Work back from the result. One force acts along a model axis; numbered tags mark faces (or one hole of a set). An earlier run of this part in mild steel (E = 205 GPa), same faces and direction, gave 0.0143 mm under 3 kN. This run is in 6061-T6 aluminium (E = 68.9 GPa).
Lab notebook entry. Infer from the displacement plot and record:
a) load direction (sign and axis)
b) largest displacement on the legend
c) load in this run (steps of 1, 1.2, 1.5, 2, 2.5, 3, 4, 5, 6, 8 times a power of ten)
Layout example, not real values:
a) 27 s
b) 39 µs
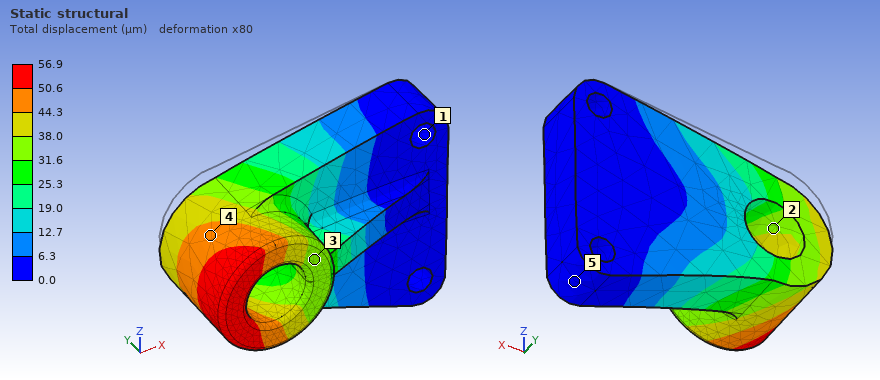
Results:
a) -Z
b) 56.9 µm
c) 4 kN
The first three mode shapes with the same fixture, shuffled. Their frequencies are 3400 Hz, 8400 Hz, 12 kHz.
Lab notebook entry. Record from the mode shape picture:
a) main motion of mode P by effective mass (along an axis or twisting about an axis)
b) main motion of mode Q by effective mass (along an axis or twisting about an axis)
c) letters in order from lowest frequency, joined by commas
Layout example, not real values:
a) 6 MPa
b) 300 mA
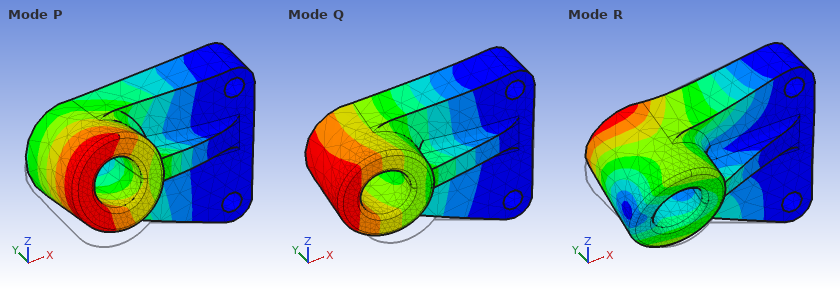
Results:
a) along Z
b) along Y
c) Q, P, R
